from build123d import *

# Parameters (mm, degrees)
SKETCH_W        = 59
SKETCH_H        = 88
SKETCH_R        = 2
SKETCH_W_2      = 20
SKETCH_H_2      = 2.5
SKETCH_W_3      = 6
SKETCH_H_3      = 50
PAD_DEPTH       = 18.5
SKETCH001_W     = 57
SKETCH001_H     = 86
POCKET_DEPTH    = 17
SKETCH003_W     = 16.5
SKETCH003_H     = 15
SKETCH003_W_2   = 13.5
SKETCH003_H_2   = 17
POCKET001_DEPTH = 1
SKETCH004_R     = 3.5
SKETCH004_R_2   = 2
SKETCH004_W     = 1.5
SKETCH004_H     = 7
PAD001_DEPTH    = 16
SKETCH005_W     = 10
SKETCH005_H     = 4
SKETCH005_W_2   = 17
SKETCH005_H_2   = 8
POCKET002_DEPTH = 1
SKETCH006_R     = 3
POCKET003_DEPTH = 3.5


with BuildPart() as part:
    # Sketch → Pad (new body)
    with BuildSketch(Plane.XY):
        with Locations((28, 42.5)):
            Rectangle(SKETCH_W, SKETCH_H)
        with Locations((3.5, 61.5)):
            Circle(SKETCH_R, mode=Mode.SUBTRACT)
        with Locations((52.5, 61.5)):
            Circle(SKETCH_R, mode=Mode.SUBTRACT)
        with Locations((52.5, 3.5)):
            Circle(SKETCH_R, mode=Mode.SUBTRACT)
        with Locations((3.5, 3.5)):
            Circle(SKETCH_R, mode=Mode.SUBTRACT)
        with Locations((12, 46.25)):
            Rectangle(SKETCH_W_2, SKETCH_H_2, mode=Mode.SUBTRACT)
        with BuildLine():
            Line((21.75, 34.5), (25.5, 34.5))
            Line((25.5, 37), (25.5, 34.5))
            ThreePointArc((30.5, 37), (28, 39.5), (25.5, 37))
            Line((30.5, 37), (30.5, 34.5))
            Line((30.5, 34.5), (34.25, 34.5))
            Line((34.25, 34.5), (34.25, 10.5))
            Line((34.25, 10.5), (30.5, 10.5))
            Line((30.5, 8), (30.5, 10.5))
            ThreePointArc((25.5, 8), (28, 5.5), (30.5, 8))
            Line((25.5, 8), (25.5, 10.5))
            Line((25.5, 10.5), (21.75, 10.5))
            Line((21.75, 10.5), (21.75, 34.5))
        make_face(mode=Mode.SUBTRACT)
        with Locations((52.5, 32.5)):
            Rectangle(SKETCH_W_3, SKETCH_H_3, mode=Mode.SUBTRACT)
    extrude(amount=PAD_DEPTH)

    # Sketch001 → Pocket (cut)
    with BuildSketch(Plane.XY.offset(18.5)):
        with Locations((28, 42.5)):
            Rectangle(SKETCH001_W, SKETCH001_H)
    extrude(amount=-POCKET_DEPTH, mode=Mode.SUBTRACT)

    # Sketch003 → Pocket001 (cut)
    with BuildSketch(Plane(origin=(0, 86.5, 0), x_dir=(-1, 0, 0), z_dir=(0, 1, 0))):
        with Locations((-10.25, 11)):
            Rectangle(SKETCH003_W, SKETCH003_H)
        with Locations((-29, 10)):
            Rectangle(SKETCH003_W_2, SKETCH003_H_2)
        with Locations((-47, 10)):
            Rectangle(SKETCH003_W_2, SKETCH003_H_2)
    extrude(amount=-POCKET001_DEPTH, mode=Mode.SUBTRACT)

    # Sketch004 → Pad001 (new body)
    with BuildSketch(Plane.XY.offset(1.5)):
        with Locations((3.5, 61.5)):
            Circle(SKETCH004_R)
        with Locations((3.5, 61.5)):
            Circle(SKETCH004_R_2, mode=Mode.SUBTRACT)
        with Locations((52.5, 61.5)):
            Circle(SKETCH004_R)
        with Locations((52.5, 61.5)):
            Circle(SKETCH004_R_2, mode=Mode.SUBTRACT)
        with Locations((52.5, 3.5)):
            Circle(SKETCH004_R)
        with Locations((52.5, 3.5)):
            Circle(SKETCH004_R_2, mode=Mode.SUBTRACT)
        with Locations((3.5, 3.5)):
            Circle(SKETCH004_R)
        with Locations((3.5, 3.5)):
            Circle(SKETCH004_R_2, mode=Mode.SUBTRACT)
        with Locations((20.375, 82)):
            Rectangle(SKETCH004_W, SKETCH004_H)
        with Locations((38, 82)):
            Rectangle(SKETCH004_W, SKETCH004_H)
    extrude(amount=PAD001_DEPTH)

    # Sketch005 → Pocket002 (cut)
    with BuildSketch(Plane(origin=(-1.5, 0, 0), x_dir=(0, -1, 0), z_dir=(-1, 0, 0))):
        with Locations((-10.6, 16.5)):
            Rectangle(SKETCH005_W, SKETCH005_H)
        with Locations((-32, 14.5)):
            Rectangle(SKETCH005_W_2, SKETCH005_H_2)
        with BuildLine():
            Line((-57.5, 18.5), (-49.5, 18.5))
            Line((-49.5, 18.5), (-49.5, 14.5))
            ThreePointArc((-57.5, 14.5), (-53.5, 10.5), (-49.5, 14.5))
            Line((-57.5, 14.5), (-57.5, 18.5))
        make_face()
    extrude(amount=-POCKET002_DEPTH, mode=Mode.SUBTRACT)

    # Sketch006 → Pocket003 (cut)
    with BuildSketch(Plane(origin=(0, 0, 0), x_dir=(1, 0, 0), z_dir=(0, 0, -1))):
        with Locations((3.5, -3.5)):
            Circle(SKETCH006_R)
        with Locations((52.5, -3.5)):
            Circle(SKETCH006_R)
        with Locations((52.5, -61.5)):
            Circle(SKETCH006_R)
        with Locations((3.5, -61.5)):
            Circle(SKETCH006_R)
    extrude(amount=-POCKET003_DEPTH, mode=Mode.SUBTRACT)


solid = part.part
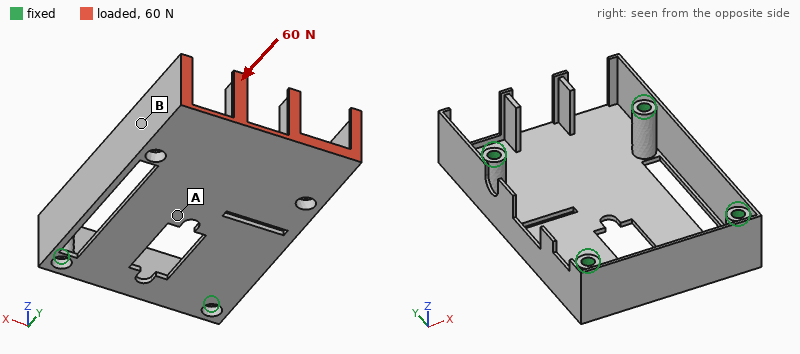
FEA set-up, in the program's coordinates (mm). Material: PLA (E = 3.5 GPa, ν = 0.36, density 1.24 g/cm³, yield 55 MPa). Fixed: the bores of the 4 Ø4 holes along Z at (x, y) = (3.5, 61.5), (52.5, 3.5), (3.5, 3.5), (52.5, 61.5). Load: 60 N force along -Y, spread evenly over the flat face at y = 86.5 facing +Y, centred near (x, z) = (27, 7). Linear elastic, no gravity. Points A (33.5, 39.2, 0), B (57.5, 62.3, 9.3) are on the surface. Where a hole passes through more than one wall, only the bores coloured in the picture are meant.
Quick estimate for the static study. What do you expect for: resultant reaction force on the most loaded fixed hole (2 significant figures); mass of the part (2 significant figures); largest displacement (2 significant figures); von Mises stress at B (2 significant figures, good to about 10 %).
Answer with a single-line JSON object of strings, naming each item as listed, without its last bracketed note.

{"resultant reaction force on the most loaded fixed hole": "19 N", "mass of the part": "15 g", "largest displacement": "1.2 mm", "von Mises stress at B": "2.4 MPa"}
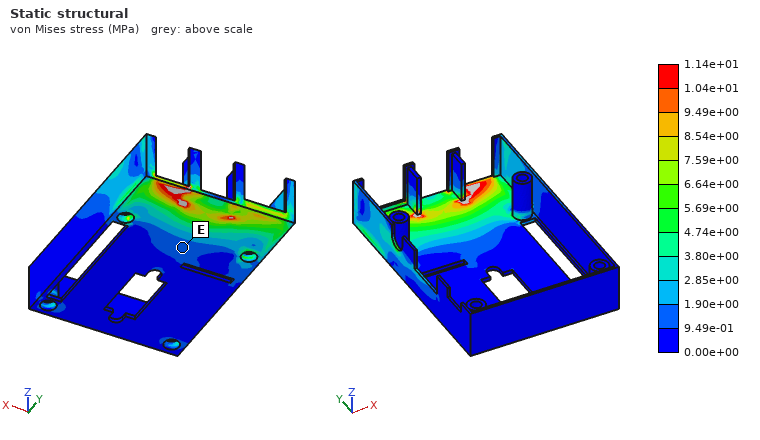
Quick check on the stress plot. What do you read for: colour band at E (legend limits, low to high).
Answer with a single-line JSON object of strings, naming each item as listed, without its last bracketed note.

{"colour band at E": "9.49e-01 to 1.90e+00 MPa"}
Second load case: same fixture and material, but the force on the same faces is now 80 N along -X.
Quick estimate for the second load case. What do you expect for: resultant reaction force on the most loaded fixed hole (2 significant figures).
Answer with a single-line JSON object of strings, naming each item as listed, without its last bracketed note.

{"resultant reaction force on the most loaded fixed hole": "54 N"}
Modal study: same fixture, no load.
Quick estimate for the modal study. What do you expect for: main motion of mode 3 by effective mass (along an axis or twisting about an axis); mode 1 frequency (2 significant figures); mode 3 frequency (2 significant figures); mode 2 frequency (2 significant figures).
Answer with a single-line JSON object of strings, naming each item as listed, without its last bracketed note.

{"main motion of mode 3 by effective mass": "along Z", "mode 1 frequency": "490 Hz", "mode 3 frequency": "620 Hz", "mode 2 frequency": "510 Hz"}
